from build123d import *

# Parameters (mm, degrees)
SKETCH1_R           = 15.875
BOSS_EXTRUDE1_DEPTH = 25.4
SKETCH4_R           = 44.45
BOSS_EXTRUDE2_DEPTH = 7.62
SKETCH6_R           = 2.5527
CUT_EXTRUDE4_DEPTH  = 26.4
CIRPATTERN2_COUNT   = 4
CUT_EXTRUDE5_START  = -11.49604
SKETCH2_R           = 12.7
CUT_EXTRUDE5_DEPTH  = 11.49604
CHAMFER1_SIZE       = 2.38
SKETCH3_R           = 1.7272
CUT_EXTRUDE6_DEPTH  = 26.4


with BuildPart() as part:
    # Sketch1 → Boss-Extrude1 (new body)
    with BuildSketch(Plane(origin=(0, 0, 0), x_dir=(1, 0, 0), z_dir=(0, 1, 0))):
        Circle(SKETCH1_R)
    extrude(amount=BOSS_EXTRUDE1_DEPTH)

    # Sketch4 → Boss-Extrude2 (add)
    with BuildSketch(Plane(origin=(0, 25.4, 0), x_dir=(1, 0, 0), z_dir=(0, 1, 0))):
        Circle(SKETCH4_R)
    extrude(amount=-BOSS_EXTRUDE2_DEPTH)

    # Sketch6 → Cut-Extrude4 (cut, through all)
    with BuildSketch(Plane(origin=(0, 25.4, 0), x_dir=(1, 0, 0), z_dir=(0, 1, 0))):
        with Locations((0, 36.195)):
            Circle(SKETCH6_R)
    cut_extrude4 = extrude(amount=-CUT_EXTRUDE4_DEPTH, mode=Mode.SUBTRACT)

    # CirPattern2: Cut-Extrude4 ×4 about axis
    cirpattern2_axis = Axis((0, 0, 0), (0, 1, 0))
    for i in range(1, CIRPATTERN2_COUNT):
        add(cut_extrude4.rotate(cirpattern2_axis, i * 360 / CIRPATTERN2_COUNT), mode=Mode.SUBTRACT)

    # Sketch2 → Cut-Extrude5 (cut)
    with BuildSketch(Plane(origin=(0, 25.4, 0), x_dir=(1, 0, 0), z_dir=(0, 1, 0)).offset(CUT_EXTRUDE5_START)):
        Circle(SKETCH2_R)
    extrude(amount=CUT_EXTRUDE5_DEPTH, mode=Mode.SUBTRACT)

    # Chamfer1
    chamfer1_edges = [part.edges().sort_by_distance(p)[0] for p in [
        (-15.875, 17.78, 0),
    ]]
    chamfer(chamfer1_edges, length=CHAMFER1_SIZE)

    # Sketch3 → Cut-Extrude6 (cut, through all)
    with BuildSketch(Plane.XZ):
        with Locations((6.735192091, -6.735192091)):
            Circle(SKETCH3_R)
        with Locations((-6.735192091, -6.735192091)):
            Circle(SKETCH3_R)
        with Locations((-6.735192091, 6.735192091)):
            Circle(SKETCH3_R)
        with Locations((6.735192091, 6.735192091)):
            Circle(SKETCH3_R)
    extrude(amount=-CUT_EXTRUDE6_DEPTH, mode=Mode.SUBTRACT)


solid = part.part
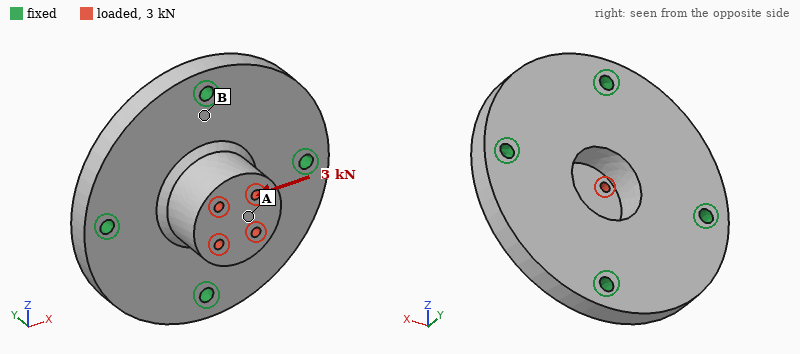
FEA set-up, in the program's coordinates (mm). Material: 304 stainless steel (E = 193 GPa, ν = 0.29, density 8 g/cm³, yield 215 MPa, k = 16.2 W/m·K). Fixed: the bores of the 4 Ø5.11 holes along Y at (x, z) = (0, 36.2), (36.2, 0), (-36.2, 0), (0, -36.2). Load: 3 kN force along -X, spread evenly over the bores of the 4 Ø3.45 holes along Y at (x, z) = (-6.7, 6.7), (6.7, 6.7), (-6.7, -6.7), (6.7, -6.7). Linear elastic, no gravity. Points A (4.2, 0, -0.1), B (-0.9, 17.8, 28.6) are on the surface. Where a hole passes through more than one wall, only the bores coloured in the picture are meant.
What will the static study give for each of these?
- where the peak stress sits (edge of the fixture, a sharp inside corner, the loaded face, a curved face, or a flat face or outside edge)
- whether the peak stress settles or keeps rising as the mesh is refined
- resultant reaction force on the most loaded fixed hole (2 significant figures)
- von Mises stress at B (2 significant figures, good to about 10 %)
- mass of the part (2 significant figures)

edge of the fixture
keeps rising
1.2 kN
8.7 MPa
440 g
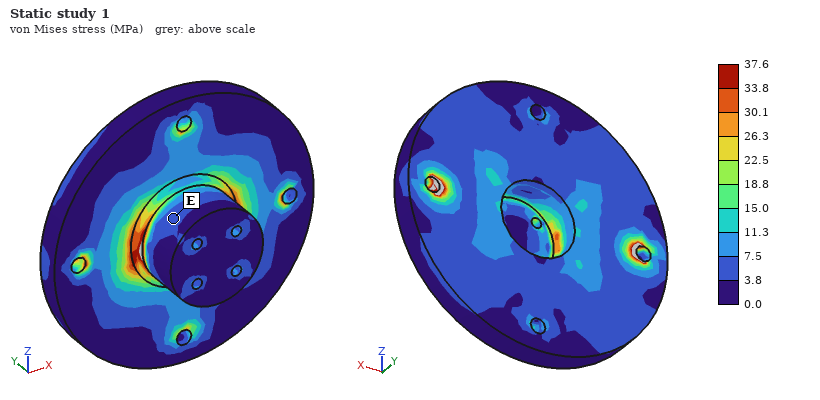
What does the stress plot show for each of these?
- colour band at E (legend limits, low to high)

3.8 to 7.5 MPa
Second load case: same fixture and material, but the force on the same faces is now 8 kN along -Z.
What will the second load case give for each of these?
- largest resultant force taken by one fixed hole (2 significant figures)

3.1 kN
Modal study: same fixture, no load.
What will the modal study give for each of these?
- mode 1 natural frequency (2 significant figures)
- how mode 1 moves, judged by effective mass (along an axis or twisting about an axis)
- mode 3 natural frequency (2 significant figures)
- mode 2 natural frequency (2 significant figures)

8400 Hz
along Y
9700 Hz
9700 Hz
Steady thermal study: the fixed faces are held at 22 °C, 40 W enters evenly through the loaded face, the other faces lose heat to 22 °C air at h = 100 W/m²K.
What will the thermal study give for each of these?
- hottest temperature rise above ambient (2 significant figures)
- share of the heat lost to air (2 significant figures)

76 K
74 %
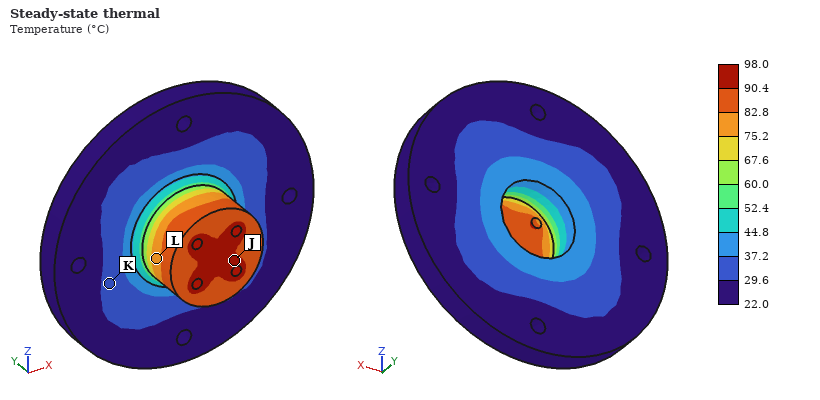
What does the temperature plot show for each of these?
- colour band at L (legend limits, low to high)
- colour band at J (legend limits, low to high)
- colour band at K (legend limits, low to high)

75.2 to 82.8 °C
90.4 to 98.0 °C
29.6 to 37.2 °C
